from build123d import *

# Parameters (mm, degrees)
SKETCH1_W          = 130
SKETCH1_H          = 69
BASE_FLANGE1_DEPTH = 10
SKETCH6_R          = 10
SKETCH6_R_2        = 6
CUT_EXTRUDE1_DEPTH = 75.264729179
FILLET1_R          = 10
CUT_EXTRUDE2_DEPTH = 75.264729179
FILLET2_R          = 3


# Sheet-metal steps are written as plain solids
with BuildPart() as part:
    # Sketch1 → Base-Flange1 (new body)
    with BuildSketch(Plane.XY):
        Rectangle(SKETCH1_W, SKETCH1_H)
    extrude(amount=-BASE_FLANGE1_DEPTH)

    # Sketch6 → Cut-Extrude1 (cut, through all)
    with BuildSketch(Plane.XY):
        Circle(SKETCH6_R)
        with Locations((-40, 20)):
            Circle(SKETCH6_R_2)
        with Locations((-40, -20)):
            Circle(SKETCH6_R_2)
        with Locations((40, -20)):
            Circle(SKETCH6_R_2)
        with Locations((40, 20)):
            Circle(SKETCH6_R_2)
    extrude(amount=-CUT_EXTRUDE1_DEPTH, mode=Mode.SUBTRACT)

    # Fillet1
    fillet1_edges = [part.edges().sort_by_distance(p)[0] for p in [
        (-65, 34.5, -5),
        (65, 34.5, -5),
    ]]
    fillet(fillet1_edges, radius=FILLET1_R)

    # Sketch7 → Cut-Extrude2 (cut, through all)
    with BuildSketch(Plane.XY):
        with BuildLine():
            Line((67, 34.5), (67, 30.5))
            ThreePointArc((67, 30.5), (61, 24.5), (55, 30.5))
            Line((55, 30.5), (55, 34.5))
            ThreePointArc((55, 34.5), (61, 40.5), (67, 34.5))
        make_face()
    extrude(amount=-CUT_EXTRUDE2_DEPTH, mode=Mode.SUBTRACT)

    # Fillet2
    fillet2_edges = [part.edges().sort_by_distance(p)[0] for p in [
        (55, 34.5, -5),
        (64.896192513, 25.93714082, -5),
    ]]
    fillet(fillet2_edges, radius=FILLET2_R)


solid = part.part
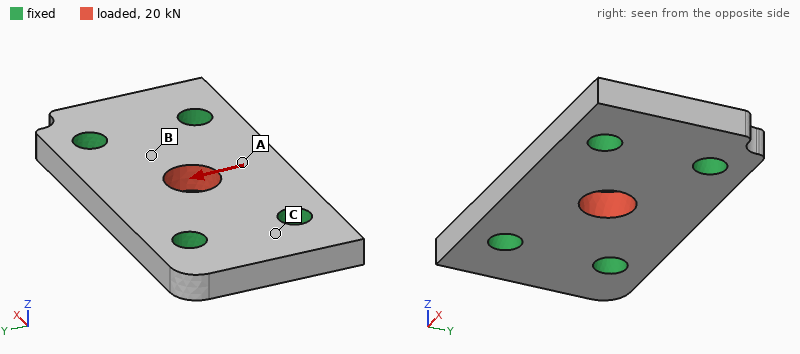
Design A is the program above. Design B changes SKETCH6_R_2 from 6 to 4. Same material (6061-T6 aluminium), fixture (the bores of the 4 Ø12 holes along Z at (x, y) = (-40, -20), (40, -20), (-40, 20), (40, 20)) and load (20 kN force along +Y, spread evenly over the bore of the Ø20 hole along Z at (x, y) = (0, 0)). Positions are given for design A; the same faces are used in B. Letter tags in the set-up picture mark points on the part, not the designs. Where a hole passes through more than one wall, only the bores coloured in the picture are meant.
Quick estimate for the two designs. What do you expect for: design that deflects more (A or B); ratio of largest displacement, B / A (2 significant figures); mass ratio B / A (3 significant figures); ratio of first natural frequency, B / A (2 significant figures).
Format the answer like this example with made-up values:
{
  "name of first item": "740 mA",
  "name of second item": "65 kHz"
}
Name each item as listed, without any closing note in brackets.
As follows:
{
  "design that deflects more": "B",
  "ratio of largest displacement, B / A": "1.1",
  "mass ratio B / A": "1.03",
  "ratio of first natural frequency, B / A": "0.87"
}
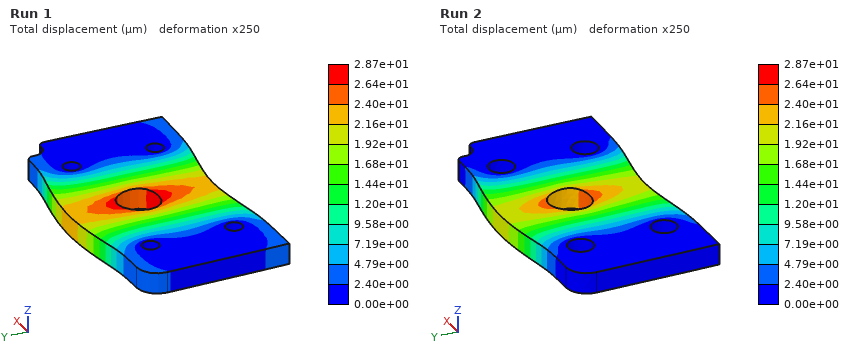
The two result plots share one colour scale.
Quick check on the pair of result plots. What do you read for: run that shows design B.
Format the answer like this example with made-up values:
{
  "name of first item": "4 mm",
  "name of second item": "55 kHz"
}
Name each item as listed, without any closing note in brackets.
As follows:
{
  "run that shows design B": "Run 1"
}
